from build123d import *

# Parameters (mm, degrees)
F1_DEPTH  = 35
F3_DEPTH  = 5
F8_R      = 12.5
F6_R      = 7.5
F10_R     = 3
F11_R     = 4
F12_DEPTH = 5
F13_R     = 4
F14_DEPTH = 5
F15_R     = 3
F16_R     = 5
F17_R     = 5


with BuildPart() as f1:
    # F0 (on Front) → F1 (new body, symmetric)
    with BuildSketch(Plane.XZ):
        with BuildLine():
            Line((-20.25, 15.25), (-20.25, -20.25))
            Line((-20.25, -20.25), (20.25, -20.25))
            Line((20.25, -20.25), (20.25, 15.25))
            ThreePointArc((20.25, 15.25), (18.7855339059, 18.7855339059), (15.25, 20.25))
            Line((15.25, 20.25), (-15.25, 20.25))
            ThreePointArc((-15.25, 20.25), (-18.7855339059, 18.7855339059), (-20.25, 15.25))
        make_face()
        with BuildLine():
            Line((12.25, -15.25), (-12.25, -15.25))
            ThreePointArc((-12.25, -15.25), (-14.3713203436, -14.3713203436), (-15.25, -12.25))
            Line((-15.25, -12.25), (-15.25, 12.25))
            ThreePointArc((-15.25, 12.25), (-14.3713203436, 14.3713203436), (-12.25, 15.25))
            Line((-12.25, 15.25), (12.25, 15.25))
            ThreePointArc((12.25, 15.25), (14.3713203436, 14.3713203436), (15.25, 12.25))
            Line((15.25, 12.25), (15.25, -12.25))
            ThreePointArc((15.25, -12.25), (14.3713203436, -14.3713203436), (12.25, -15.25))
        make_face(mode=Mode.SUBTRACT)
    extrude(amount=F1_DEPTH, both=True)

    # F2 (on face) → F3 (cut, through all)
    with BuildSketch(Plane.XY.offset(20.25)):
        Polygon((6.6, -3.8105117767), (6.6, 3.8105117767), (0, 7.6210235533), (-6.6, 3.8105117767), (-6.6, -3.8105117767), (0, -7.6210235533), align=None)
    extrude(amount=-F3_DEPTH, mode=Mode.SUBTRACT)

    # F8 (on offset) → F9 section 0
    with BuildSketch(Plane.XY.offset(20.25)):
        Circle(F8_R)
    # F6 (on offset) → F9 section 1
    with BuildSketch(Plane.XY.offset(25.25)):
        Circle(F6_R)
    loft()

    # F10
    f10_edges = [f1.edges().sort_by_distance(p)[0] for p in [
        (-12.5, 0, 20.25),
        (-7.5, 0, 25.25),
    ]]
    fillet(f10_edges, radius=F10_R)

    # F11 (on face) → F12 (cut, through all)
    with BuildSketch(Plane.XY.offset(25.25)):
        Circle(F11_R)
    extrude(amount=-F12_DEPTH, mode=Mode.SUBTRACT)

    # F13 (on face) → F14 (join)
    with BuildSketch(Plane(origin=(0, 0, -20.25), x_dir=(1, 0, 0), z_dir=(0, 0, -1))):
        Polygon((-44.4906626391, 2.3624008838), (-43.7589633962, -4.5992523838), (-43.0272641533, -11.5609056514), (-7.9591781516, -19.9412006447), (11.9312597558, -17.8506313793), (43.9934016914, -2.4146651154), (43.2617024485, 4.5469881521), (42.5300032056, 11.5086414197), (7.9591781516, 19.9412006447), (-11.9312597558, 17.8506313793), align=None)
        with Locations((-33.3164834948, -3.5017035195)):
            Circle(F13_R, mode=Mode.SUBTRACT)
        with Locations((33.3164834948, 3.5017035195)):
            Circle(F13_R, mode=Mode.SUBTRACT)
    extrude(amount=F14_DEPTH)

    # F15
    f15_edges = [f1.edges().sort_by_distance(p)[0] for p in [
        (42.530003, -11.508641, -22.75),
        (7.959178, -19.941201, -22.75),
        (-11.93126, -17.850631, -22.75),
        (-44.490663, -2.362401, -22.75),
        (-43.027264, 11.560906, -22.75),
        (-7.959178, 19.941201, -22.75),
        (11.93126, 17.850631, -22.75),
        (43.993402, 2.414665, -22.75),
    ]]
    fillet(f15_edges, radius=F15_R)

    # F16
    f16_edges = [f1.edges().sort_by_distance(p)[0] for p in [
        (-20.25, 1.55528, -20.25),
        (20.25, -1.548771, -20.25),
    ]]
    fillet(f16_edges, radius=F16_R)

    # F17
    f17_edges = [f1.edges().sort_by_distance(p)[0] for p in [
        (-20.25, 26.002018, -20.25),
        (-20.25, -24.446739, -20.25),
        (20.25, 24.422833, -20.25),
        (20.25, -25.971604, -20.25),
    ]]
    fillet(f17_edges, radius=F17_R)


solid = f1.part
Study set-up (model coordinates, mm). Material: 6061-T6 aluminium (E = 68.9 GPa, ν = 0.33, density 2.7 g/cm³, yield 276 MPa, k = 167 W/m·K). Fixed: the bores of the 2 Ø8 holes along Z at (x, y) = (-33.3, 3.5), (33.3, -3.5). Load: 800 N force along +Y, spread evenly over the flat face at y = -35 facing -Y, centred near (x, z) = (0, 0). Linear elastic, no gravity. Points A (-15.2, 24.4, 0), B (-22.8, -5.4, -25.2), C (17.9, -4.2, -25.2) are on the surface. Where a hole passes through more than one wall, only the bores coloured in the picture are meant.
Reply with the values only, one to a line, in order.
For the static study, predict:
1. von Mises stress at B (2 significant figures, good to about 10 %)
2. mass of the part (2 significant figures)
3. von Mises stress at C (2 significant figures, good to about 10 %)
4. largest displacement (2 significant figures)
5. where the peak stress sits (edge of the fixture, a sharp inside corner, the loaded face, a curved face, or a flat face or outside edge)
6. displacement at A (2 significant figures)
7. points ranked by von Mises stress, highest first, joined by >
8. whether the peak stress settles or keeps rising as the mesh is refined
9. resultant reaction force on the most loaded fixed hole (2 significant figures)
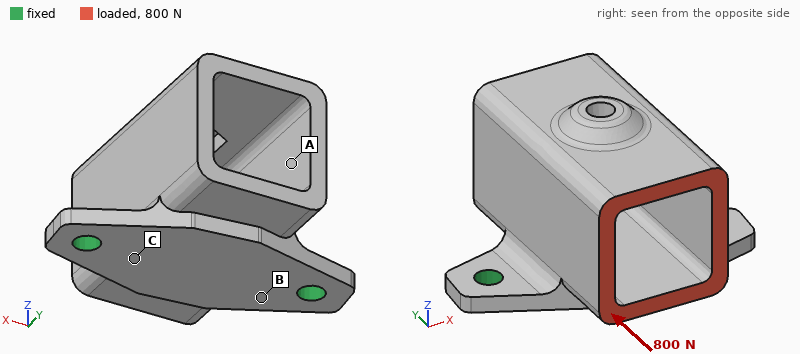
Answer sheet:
25 MPa
170 g
14 MPa
0.14 mm
edge of the fixture
0.081 mm
B > C > A
keeps rising
400 N
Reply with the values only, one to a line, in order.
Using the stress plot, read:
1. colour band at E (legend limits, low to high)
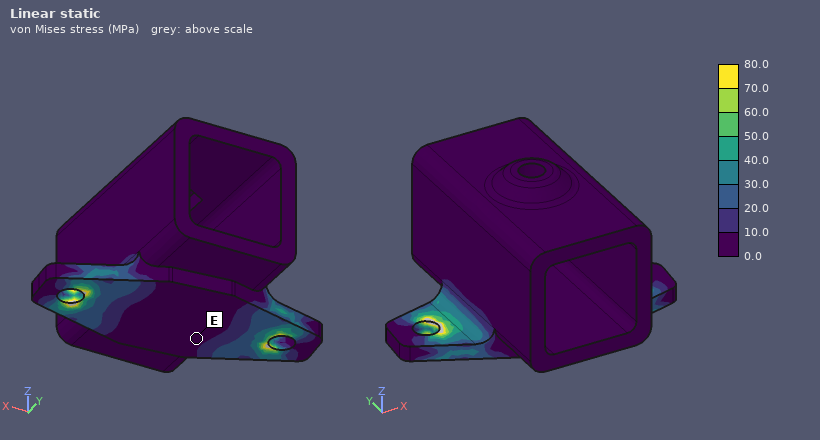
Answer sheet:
0.0 to 10.0 MPa
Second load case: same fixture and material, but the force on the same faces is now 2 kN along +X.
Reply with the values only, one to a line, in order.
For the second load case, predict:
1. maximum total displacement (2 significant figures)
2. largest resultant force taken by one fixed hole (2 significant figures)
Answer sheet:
0.12 mm
1.8 kN
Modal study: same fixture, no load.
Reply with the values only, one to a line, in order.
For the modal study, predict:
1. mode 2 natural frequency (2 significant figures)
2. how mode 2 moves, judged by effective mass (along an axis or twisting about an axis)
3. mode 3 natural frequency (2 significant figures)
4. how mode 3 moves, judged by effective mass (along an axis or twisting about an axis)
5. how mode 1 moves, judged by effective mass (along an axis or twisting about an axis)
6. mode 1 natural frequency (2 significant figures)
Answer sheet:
2800 Hz
along X
4500 Hz
along Z
along Y
1100 Hz
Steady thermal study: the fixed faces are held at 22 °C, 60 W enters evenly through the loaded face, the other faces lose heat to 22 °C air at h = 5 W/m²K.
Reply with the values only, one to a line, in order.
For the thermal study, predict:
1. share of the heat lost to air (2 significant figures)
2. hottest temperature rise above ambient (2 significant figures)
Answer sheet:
4.6 %
43 K
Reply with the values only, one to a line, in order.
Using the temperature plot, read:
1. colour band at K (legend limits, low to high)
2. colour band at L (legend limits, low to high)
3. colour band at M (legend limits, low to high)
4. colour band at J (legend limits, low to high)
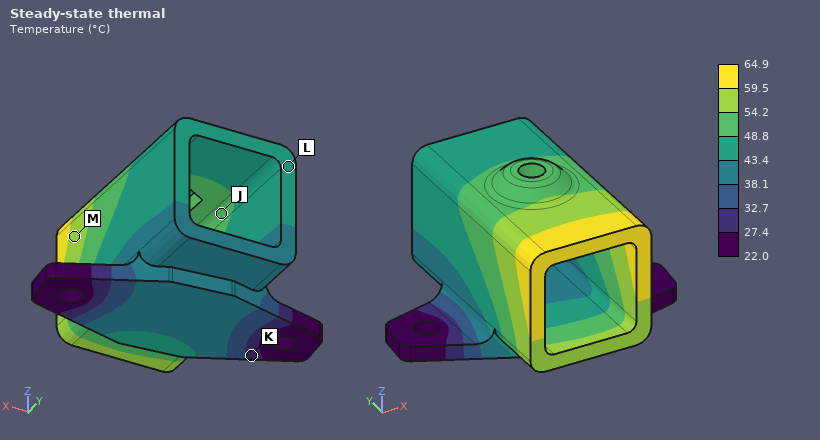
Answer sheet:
27.4 to 32.7 °C
43.4 to 48.8 °C
54.2 to 59.5 °C
48.8 to 54.2 °C
